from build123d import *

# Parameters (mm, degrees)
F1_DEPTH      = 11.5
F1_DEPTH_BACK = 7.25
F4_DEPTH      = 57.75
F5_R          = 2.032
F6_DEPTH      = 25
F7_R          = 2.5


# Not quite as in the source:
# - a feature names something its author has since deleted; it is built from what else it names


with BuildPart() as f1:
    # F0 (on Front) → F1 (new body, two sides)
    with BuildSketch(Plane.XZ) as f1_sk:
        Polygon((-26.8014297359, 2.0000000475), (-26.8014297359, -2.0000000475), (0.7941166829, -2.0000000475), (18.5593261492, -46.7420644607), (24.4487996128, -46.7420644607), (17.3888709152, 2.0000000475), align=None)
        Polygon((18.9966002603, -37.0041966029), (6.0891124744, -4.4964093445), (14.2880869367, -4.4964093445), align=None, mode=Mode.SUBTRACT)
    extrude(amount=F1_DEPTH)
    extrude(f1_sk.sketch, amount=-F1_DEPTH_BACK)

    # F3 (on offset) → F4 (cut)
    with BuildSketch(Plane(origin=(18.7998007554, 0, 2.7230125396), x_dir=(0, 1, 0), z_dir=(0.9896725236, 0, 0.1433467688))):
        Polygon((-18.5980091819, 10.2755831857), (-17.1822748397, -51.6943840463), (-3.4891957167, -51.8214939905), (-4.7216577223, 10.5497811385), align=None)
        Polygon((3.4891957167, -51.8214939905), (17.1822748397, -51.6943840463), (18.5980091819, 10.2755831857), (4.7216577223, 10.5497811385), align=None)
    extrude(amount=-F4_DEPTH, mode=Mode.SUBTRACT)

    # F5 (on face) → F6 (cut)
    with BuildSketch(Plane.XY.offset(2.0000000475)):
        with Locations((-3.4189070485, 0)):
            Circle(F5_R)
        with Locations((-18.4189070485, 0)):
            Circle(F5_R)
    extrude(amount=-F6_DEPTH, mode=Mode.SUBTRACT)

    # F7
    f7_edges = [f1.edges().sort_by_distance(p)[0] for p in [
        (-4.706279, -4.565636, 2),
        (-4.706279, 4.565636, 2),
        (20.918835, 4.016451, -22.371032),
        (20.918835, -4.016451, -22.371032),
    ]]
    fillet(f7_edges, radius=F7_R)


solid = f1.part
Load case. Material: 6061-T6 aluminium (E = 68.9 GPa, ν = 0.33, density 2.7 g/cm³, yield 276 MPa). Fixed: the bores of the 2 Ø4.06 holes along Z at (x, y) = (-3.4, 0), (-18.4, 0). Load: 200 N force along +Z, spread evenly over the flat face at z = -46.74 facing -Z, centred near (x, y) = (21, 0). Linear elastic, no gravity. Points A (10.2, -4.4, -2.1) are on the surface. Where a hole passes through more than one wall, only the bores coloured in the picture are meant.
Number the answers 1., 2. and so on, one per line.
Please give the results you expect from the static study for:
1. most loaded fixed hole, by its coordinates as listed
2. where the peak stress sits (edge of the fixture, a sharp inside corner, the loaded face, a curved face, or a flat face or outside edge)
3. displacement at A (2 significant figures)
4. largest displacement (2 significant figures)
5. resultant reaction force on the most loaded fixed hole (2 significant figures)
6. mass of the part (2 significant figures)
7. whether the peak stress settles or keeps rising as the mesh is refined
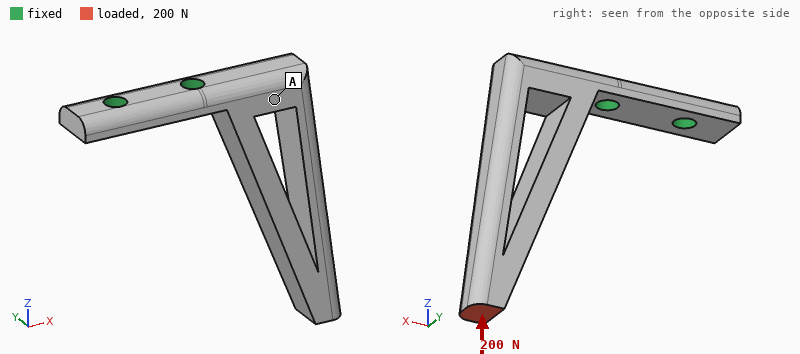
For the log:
1. (-3.4, 0)
2. edge of the fixture
3. 0.076 mm
4. 0.43 mm
5. 210 N
6. 12 g
7. keeps rising
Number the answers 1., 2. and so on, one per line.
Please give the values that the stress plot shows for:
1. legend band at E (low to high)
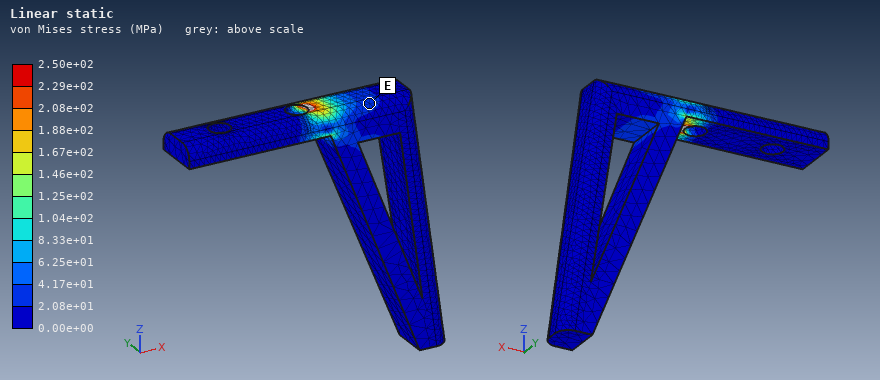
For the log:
1. 2.08e+01 to 4.17e+01 MPa
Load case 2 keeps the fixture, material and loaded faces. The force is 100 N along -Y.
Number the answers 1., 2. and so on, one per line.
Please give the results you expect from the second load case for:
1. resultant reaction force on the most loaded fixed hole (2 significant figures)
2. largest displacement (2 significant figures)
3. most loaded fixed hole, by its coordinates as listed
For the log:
1. 130 N
2. 0.43 mm
3. (-3.4, 0)
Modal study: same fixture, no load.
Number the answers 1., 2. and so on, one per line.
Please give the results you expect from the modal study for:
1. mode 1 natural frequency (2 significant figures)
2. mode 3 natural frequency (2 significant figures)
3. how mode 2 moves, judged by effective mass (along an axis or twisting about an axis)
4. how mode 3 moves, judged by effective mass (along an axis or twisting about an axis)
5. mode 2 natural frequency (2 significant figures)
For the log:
1. 1300 Hz
2. 7600 Hz
3. along Y
4. along Y
5. 1700 Hz
